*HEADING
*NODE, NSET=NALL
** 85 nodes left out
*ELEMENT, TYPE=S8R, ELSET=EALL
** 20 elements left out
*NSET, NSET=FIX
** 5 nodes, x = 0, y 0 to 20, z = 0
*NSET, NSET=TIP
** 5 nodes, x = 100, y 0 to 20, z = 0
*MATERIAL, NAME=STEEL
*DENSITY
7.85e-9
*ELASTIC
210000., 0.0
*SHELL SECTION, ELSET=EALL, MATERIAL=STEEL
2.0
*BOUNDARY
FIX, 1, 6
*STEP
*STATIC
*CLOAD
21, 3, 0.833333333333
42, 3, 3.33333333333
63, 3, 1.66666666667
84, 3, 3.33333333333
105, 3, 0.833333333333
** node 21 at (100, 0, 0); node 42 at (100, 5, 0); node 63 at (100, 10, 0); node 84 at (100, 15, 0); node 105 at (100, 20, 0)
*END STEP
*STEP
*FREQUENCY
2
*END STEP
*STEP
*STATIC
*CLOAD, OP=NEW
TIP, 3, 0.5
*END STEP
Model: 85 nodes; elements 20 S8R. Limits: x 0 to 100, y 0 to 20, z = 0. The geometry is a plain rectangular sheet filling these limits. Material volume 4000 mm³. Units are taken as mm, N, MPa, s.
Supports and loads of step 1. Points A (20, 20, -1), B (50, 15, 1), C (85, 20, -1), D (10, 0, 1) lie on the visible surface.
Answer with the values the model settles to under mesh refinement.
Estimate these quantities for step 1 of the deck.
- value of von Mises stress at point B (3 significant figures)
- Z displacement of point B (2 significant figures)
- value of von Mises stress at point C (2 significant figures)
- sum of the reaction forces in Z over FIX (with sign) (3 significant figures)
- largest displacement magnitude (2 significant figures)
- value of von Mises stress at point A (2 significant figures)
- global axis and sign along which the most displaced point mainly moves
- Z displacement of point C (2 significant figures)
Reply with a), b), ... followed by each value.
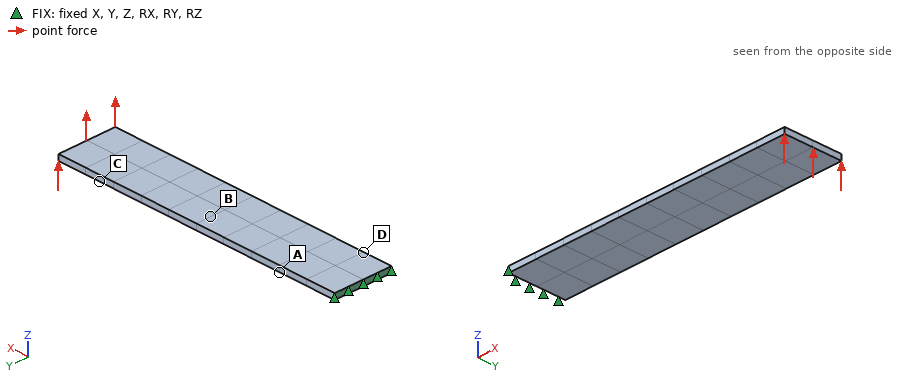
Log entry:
a) 37.5 MPa
b) 0.37 mm
c) 11 MPa
d) -10.0 N
e) 1.2 mm
f) 60 MPa
g) +Z
h) 0.92 mm
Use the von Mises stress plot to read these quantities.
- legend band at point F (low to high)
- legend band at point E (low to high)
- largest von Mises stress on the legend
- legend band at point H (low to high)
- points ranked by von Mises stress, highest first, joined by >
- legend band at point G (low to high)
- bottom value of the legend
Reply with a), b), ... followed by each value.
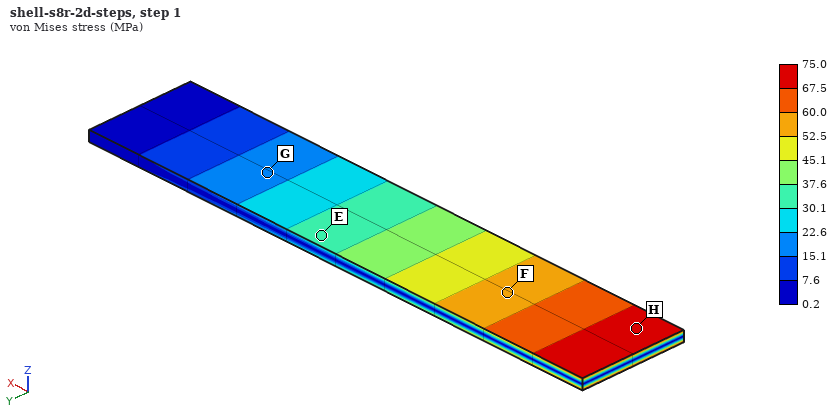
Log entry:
a) 52.5 to 60.0 MPa
b) 30.1 to 37.6 MPa
c) 75.0 MPa
d) 67.5 to 75.0 MPa
e) H > F > E > G
f) 15.1 to 22.6 MPa
g) 0.2 MPa
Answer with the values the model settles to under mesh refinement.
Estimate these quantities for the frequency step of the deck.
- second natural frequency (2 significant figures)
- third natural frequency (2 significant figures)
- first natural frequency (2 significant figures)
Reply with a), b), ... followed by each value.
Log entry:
a) 1000 Hz
b) 1600 Hz
c) 170 Hz
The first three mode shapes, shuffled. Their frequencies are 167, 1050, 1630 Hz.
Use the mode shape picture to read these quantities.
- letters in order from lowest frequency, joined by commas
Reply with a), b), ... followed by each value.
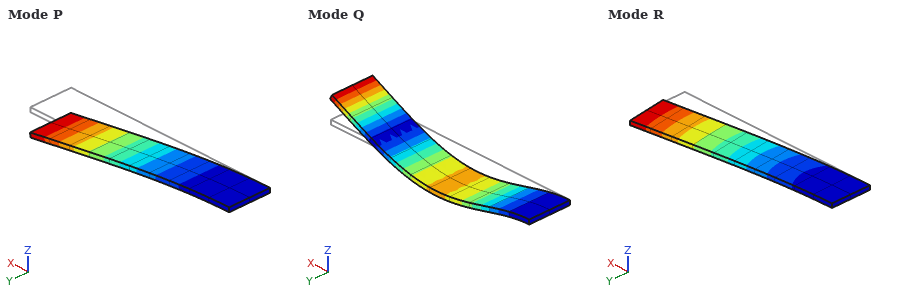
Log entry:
a) P, Q, R
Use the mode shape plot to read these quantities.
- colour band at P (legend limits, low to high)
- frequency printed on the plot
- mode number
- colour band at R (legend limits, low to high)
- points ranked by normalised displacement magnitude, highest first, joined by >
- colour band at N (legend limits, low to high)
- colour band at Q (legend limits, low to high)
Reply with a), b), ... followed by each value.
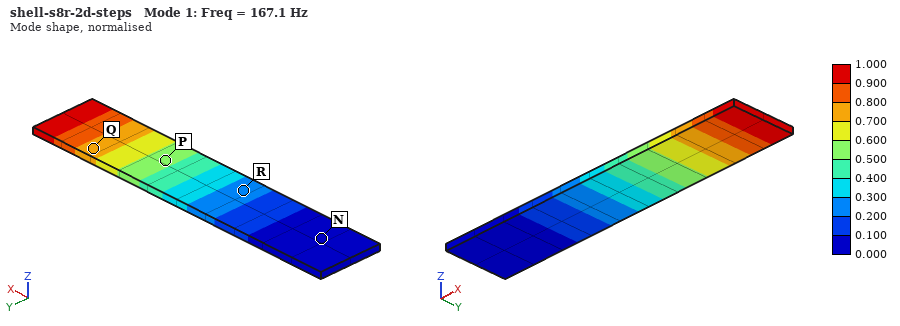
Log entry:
a) 0.500 to 0.600
b) 167.1 Hz
c) 1
d) 0.200 to 0.300
e) Q > P > R > N
f) 0.000 to 0.100
g) 0.700 to 0.800
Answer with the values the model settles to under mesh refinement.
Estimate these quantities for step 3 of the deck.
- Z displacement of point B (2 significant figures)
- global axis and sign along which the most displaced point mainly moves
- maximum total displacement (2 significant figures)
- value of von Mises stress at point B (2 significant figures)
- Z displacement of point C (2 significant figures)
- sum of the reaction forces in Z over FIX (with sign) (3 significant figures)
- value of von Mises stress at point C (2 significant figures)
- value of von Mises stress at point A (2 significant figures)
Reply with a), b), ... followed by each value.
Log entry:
a) 0.093 mm
b) +Z
c) 0.30 mm
d) 9.4 MPa
e) 0.23 mm
f) -2.50 N
g) 2.8 MPa
h) 15 MPa
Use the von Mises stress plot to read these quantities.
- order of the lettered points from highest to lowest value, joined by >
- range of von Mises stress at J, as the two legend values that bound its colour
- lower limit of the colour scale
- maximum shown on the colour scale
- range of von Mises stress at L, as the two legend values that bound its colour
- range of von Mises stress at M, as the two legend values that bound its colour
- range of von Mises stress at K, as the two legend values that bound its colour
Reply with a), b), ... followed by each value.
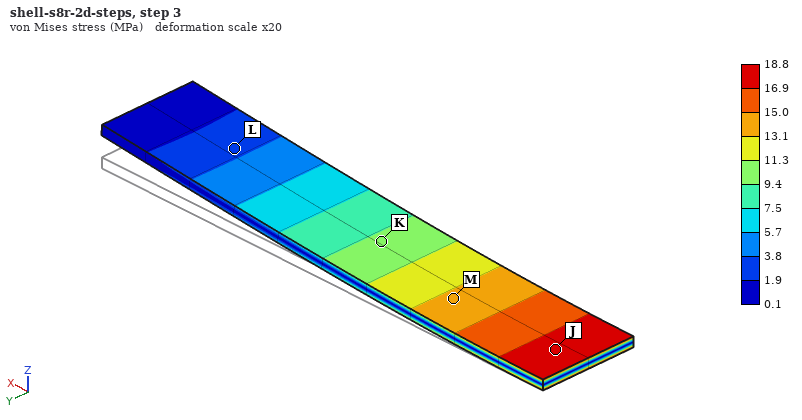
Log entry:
a) J > M > K > L
b) 16.9 to 18.8 MPa
c) 0.1 MPa
d) 18.8 MPa
e) 1.9 to 3.8 MPa
f) 13.1 to 15.0 MPa
g) 9.4 to 11.3 MPa
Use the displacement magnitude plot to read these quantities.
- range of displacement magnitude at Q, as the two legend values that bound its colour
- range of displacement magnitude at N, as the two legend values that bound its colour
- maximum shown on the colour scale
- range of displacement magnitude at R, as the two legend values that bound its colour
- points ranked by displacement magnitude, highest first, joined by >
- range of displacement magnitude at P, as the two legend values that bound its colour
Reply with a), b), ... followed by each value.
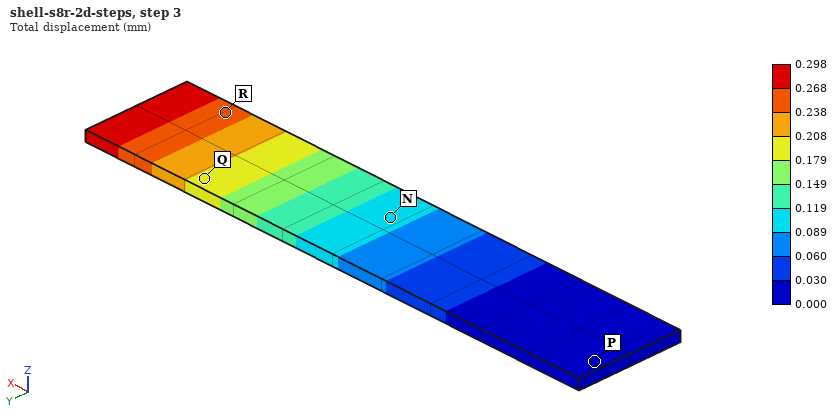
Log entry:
a) 0.179 to 0.208 mm
b) 0.089 to 0.119 mm
c) 0.298 mm
d) 0.238 to 0.268 mm
e) R > Q > N > P
f) 0.000 to 0.030 mm
